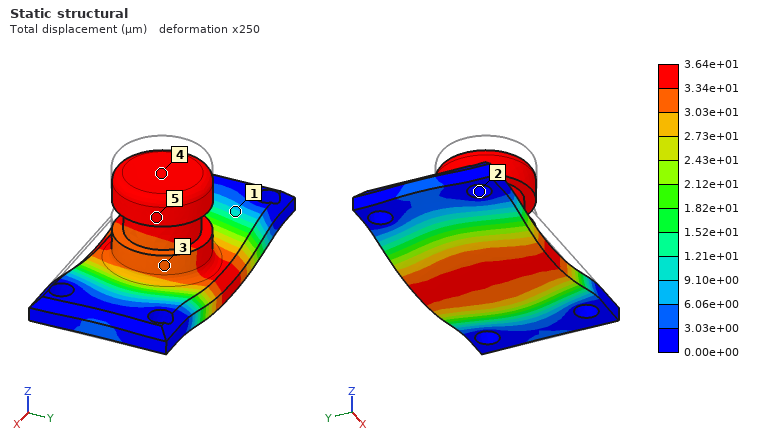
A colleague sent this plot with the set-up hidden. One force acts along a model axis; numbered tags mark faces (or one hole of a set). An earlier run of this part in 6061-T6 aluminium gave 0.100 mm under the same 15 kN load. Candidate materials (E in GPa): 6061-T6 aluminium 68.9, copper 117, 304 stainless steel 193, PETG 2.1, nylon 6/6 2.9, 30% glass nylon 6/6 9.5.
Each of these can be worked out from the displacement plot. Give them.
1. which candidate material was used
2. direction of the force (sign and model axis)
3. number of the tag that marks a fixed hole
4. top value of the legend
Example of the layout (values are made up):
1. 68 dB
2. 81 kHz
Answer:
1. 304 stainless steel
2. -Z
3. 2
4. 3.64e+01 µm
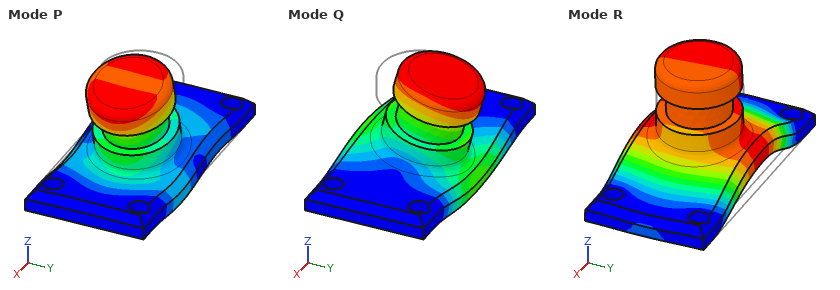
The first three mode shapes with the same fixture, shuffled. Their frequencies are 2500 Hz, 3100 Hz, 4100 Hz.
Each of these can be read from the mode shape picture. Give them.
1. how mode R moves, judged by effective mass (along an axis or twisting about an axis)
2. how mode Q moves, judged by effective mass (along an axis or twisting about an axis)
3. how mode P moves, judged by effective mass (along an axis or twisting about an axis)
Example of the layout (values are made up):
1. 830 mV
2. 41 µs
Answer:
1. along Z
2. along Y
3. along X
